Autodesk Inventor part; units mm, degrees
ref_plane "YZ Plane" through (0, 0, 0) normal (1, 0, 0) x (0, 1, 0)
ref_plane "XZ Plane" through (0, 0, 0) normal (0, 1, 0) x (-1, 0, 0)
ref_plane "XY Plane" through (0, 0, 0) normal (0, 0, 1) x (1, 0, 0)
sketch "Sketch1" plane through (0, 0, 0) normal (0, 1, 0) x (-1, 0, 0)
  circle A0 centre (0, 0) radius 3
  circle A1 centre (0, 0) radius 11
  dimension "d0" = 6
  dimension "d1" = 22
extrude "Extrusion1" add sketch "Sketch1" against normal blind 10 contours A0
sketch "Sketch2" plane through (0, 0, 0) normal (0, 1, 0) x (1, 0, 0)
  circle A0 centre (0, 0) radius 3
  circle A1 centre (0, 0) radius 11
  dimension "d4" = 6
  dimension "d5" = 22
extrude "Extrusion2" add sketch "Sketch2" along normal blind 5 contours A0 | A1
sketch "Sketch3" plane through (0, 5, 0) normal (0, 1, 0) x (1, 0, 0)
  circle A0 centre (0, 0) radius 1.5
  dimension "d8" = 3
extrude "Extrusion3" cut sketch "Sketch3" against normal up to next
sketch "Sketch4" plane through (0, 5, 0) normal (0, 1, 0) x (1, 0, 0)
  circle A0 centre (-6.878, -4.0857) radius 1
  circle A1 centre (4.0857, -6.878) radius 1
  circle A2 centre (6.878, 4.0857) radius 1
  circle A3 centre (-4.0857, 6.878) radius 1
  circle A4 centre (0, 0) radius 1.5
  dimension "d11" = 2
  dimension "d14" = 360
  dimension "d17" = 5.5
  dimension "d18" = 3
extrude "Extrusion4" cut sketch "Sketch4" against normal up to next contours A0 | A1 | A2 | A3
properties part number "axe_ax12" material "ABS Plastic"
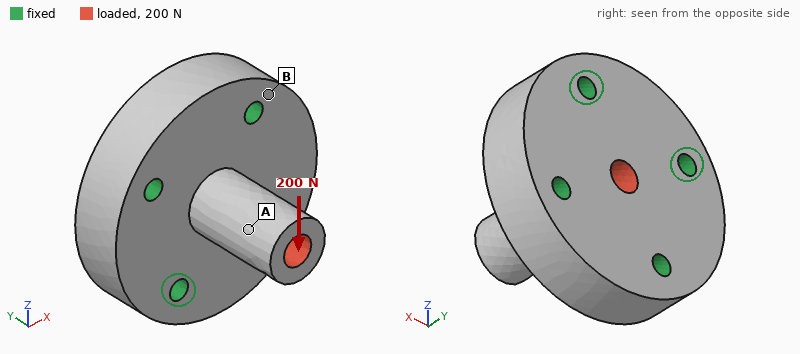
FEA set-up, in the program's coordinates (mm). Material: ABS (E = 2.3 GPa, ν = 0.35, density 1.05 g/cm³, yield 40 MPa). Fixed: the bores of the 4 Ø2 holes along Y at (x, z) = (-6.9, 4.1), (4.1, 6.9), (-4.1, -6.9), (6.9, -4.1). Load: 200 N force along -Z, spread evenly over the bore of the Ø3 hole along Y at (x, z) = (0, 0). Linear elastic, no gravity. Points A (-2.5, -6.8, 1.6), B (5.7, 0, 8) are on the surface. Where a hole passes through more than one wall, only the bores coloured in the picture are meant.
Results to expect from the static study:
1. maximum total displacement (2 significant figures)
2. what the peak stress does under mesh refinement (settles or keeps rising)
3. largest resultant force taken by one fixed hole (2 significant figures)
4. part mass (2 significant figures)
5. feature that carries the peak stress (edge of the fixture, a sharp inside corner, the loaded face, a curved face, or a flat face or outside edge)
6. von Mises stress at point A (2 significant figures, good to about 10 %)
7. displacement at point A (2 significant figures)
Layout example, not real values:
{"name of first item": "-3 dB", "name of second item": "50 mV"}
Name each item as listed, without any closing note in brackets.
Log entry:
{"maximum total displacement": "0.28 mm", "what the peak stress does under mesh refinement": "keeps rising", "largest resultant force taken by one fixed hole": "84 N", "part mass": "2.1 g", "feature that carries the peak stress": "a sharp inside corner", "von Mises stress at point A": "5.0 MPa", "displacement at point A": "0.19 mm"}
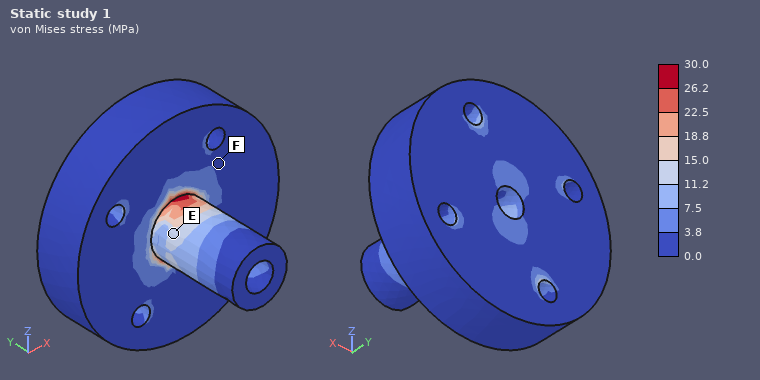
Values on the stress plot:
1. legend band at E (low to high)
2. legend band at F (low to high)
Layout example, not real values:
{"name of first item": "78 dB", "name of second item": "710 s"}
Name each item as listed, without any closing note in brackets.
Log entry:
{"legend band at E": "11.2 to 15.0 MPa", "legend band at F": "0.0 to 3.8 MPa"}
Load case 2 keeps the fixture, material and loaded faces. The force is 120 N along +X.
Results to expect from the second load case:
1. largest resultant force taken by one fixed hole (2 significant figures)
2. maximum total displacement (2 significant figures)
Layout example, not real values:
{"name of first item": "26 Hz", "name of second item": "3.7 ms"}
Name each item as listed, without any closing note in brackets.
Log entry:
{"largest resultant force taken by one fixed hole": "50 N", "maximum total displacement": "0.17 mm"}
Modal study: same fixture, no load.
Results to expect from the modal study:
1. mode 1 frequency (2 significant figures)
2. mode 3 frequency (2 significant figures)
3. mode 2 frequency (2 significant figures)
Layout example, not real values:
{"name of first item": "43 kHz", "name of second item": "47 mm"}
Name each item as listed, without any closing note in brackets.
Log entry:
{"mode 1 frequency": "8800 Hz", "mode 3 frequency": "21 kHz", "mode 2 frequency": "8800 Hz"}
